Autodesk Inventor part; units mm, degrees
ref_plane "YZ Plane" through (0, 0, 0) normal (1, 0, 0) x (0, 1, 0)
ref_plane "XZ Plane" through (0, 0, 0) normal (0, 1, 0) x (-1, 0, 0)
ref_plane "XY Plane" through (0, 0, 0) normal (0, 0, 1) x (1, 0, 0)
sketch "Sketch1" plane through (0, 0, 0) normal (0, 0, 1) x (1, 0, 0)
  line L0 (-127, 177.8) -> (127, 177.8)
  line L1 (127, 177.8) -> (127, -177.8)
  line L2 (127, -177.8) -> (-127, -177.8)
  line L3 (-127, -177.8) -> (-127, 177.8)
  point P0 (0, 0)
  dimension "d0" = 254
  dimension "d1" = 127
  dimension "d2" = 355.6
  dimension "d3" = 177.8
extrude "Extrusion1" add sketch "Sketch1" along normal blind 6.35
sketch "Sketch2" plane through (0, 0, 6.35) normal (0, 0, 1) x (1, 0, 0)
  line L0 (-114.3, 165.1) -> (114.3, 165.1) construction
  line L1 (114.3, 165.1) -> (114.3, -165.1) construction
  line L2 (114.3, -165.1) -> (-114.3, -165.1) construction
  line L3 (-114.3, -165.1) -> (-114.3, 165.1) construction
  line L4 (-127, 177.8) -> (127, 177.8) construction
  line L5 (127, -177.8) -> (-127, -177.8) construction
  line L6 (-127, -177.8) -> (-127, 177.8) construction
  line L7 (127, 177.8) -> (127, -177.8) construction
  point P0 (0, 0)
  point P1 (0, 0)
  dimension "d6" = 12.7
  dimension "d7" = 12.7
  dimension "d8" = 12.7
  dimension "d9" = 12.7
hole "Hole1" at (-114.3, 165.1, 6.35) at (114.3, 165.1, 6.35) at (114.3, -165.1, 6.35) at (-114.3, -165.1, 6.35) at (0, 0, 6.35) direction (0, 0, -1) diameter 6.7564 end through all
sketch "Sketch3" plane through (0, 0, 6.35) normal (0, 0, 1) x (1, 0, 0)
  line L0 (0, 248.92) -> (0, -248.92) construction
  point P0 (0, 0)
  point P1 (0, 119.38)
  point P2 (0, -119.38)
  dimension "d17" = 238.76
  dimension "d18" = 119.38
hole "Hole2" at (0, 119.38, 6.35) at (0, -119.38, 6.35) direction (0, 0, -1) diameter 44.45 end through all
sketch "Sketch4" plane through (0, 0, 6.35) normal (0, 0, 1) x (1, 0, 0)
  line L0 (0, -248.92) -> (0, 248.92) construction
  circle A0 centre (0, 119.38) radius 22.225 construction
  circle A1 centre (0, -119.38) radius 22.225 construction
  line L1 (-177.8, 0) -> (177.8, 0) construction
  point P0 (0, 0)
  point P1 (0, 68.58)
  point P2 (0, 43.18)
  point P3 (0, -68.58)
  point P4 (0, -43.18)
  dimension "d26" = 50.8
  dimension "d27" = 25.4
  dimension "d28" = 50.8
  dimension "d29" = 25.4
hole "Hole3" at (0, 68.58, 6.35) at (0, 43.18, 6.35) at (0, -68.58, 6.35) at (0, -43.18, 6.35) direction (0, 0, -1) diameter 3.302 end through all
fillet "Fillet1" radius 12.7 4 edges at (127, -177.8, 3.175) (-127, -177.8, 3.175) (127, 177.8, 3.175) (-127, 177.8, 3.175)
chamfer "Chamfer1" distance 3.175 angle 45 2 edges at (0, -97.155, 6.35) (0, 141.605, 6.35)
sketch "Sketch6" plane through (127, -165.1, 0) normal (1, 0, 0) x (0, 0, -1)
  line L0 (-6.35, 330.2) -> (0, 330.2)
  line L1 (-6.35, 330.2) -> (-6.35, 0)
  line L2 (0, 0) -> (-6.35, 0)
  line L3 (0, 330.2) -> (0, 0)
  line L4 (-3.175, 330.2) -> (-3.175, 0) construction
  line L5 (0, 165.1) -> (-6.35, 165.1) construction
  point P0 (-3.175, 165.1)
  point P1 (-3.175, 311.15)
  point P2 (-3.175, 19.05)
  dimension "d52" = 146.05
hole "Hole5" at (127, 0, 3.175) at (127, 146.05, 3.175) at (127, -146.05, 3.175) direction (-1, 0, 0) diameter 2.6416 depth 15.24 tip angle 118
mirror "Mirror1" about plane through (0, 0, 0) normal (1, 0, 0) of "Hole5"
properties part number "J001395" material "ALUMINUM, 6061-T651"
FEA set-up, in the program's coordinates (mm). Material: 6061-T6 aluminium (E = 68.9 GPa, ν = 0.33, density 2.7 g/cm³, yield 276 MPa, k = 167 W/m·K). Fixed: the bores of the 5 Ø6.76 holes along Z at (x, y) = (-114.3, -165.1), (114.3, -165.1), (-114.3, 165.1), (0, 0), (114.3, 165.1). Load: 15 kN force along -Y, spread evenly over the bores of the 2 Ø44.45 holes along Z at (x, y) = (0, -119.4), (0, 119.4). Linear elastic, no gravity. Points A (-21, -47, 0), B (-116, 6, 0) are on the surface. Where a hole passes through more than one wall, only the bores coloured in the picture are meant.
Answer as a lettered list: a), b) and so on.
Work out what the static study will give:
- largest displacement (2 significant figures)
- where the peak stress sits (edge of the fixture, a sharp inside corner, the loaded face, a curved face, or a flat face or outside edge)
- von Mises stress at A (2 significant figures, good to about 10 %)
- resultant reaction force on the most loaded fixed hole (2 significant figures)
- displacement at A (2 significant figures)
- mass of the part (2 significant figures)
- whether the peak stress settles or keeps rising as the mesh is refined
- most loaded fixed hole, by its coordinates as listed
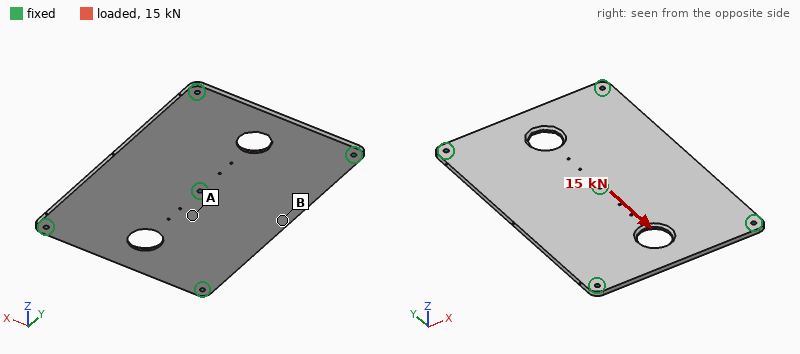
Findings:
a) 81 µm
b) edge of the fixture
c) 9.2 MPa
d) 6.5 kN
e) 14 µm
f) 1.5 kg
g) keeps rising
h) (0, 0)
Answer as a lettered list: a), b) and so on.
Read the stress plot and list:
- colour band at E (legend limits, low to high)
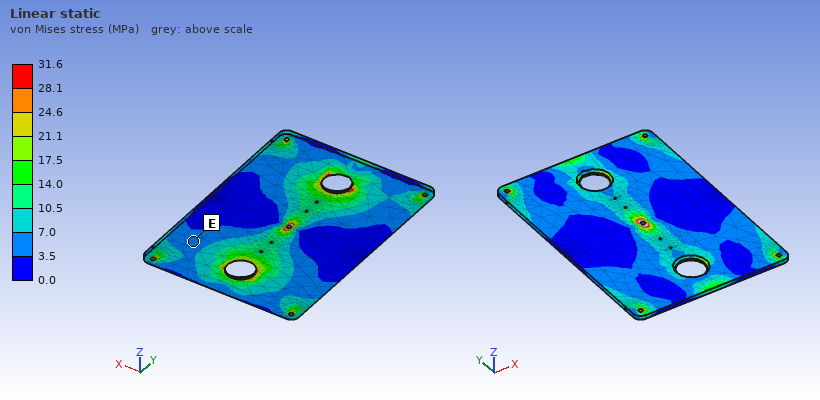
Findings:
a) 3.5 to 7.0 MPa
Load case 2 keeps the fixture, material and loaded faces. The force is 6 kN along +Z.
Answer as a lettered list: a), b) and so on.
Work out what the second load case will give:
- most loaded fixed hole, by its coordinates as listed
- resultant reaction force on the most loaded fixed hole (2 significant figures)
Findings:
a) (0, 0)
b) 2.5 kN
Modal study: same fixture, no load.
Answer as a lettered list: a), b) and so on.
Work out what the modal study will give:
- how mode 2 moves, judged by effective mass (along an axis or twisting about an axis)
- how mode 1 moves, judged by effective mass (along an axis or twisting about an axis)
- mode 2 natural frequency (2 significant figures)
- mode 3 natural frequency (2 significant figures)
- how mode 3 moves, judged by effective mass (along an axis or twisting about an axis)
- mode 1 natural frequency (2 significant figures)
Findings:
a) along Z
b) twisting about Y
c) 500 Hz
d) 590 Hz
e) twisting about X
f) 440 Hz
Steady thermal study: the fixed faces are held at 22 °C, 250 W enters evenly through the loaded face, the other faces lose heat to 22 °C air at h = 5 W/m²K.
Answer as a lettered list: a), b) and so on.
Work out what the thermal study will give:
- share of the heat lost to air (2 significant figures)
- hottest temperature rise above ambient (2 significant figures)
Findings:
a) 12 %
b) 67 K
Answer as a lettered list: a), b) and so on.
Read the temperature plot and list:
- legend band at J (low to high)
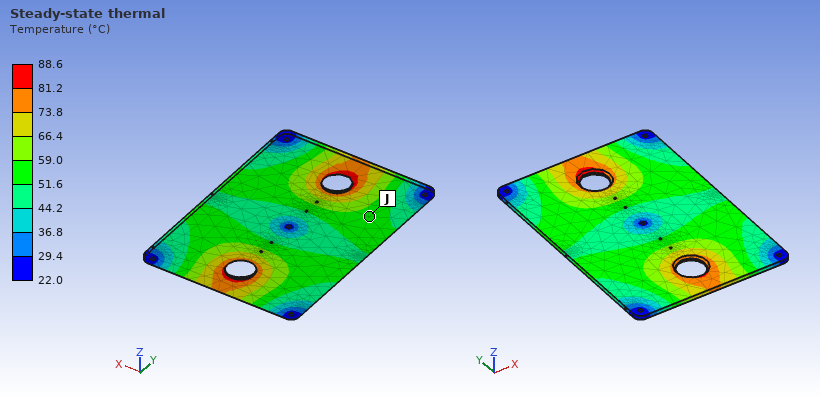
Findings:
a) 51.6 to 59.0 °C
